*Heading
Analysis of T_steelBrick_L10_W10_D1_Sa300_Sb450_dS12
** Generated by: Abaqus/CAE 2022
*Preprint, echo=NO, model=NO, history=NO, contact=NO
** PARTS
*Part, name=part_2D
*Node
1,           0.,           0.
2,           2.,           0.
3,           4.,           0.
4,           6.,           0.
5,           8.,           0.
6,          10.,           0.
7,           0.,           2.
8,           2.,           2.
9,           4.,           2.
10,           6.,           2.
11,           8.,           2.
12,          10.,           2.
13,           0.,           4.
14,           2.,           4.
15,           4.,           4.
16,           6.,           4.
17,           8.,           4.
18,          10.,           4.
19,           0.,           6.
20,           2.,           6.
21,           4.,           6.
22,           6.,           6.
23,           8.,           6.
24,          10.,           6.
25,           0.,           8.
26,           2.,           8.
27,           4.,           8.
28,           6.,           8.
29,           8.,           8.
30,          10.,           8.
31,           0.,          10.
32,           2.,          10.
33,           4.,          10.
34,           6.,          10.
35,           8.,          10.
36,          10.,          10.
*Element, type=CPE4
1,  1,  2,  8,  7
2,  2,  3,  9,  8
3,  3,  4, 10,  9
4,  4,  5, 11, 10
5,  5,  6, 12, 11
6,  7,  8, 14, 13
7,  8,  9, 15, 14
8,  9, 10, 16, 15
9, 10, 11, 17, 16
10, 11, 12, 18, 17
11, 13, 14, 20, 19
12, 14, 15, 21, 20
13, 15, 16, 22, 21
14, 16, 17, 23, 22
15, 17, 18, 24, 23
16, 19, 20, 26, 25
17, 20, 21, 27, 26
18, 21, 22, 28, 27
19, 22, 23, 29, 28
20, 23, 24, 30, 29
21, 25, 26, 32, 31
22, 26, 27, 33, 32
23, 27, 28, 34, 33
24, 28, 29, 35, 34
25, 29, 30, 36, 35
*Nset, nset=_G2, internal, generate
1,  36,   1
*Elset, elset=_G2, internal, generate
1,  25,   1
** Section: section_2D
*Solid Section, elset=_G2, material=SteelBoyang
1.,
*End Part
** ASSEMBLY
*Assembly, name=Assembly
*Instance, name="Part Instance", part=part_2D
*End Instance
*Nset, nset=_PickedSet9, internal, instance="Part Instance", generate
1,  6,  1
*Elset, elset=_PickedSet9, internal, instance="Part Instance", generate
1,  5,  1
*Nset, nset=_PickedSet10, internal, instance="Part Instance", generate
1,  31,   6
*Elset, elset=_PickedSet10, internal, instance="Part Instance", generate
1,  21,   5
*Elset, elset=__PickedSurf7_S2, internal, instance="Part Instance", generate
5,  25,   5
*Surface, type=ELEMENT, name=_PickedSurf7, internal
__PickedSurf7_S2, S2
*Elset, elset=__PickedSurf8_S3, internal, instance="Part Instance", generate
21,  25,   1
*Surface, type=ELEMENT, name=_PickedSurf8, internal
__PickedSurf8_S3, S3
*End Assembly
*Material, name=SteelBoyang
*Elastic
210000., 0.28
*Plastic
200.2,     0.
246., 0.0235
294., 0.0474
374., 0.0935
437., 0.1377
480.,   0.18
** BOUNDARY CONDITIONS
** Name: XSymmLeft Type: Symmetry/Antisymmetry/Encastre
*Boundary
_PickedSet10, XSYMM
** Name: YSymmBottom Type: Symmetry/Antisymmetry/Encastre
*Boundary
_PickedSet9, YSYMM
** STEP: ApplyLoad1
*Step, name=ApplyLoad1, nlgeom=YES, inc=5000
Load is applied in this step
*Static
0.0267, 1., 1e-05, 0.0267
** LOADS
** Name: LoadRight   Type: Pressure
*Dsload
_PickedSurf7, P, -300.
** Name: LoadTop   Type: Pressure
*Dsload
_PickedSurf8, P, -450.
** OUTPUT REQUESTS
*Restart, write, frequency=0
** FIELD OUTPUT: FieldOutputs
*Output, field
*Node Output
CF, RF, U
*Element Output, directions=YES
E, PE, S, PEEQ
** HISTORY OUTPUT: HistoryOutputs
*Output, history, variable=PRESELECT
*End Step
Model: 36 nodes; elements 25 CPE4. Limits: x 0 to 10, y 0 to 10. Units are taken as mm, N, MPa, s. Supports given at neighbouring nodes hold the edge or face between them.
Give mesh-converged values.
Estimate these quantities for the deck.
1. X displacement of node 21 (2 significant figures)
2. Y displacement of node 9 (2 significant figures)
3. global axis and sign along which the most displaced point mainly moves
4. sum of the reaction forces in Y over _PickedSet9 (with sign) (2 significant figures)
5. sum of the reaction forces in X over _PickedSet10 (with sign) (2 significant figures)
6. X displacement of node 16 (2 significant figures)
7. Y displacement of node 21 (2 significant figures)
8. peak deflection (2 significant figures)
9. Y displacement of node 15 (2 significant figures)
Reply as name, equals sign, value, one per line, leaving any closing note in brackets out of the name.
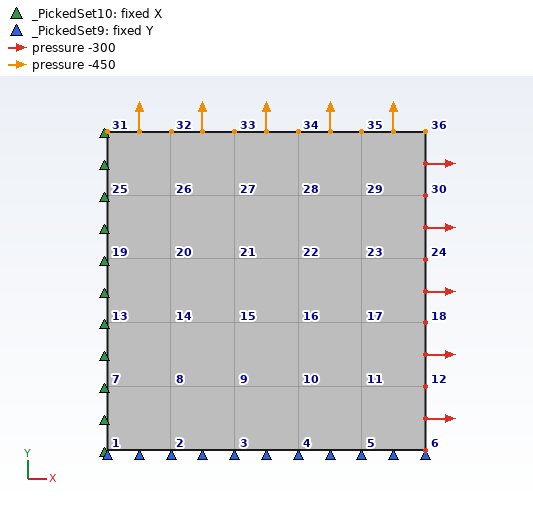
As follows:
X displacement of node 21 = 0.0021 mm
Y displacement of node 9 = 0.0030 mm
global axis and sign along which the most displaced point mainly moves = +Y
sum of the reaction forces in Y over _PickedSet9 (with sign) = -4500 N
sum of the reaction forces in X over _PickedSet10 (with sign) = -3000 N
X displacement of node 16 = 0.0031 mm
Y displacement of node 21 = 0.0091 mm
peak deflection = 0.016 mm
Y displacement of node 15 = 0.0061 mm
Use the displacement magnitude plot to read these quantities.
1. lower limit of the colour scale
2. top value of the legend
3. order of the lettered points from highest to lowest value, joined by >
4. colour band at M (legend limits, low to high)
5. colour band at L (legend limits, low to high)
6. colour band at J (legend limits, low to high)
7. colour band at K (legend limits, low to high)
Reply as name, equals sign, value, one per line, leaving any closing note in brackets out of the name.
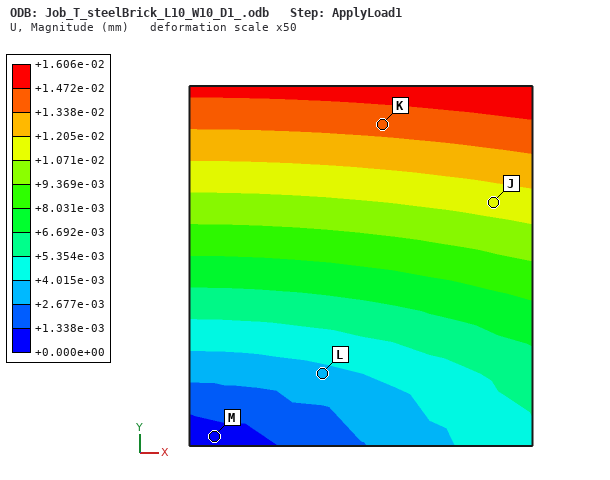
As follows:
lower limit of the colour scale = +0.000e+00 mm
top value of the legend = +1.606e-02 mm
order of the lettered points from highest to lowest value, joined by > = K > J > L > M
colour band at M = +0.000e+00 to +1.338e-03 mm
colour band at L = +2.677e-03 to +4.015e-03 mm
colour band at J = +1.071e-02 to +1.205e-02 mm
colour band at K = +1.338e-02 to +1.472e-02 mm
